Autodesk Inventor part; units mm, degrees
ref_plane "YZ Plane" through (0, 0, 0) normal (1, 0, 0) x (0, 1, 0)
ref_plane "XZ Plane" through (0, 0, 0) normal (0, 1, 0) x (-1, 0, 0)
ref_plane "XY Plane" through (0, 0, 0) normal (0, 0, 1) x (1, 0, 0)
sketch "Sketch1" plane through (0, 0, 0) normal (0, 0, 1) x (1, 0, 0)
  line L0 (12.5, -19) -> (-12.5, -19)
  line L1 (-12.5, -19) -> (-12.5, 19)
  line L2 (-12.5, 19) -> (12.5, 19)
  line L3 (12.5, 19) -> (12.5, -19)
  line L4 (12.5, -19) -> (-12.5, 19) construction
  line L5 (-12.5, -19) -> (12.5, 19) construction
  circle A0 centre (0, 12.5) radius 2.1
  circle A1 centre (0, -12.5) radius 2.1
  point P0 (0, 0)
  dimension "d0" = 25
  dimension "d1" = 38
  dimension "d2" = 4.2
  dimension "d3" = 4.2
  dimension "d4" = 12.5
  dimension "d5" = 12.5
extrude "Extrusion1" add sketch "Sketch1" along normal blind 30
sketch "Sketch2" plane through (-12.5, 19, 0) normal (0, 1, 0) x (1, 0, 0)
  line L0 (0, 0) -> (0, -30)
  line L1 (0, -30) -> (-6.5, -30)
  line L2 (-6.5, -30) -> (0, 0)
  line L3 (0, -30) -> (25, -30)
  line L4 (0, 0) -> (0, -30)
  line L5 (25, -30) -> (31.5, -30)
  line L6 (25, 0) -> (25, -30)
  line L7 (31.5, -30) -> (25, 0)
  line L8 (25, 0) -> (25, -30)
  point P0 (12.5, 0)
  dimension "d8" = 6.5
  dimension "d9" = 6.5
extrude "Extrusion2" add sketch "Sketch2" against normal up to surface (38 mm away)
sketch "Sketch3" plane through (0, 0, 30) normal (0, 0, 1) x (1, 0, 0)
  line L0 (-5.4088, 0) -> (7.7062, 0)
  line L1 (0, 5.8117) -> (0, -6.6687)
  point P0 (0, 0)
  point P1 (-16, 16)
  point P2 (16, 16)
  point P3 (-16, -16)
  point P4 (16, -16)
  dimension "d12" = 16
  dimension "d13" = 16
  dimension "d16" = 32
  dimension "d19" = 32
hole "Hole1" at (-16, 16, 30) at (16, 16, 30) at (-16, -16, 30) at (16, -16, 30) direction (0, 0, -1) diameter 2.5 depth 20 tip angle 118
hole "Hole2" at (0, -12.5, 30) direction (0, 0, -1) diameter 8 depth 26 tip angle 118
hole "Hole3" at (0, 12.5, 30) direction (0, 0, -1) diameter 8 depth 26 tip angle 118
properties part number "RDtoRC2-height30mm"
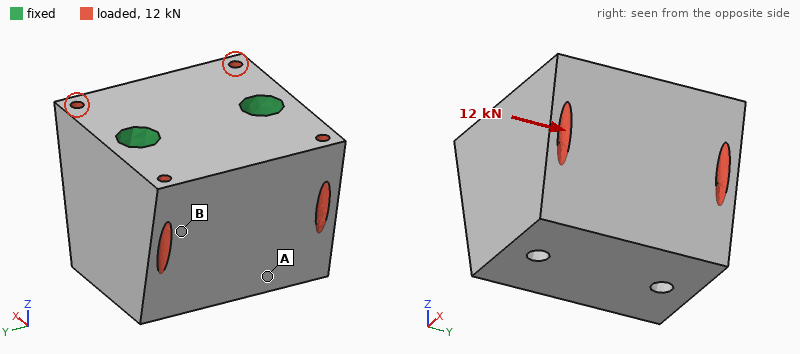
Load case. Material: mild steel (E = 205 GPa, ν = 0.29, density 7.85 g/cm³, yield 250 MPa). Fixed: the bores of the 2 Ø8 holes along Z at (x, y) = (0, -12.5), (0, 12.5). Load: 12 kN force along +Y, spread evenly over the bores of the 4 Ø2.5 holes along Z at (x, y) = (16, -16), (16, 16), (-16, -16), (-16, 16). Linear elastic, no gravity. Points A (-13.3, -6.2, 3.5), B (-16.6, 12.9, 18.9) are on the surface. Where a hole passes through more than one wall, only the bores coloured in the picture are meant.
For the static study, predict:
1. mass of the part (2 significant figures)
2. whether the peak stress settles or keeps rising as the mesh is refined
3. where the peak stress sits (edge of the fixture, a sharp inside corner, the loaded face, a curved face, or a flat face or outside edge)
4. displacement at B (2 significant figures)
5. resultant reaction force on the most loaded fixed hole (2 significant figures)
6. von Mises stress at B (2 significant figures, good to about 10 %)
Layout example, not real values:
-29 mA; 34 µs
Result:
260 g; keeps rising; a sharp inside corner; 2.1 µm; 6.2 kN; 30 MPa
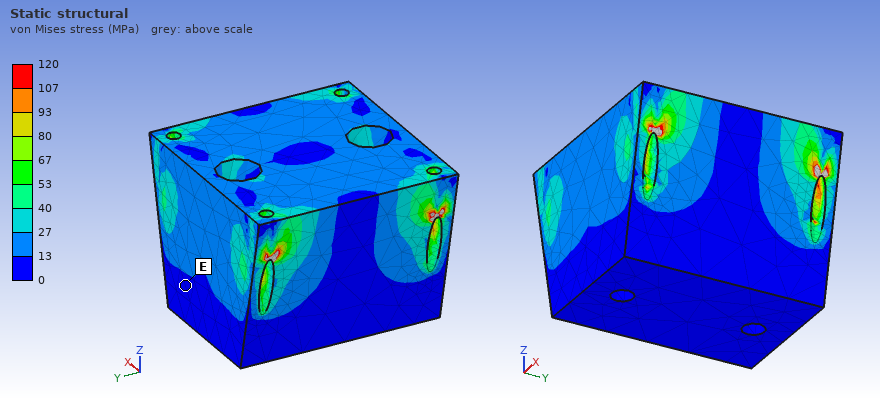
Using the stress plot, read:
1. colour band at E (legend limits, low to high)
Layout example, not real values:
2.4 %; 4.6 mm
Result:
0 to 13 MPa
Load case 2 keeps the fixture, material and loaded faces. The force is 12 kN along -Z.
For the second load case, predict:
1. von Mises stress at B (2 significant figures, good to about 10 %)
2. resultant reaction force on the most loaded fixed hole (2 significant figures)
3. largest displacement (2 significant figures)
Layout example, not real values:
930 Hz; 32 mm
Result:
45 MPa; 6.0 kN; 5.4 µm
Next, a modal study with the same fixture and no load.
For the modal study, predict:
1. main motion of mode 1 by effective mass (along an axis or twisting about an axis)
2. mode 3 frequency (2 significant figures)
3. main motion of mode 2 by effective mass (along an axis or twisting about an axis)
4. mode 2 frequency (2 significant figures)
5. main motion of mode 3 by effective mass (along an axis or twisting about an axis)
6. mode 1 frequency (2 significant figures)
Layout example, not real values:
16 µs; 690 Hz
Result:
twisting about Y; 47 kHz; along Z; 44 kHz; twisting about Z; 40 kHz
